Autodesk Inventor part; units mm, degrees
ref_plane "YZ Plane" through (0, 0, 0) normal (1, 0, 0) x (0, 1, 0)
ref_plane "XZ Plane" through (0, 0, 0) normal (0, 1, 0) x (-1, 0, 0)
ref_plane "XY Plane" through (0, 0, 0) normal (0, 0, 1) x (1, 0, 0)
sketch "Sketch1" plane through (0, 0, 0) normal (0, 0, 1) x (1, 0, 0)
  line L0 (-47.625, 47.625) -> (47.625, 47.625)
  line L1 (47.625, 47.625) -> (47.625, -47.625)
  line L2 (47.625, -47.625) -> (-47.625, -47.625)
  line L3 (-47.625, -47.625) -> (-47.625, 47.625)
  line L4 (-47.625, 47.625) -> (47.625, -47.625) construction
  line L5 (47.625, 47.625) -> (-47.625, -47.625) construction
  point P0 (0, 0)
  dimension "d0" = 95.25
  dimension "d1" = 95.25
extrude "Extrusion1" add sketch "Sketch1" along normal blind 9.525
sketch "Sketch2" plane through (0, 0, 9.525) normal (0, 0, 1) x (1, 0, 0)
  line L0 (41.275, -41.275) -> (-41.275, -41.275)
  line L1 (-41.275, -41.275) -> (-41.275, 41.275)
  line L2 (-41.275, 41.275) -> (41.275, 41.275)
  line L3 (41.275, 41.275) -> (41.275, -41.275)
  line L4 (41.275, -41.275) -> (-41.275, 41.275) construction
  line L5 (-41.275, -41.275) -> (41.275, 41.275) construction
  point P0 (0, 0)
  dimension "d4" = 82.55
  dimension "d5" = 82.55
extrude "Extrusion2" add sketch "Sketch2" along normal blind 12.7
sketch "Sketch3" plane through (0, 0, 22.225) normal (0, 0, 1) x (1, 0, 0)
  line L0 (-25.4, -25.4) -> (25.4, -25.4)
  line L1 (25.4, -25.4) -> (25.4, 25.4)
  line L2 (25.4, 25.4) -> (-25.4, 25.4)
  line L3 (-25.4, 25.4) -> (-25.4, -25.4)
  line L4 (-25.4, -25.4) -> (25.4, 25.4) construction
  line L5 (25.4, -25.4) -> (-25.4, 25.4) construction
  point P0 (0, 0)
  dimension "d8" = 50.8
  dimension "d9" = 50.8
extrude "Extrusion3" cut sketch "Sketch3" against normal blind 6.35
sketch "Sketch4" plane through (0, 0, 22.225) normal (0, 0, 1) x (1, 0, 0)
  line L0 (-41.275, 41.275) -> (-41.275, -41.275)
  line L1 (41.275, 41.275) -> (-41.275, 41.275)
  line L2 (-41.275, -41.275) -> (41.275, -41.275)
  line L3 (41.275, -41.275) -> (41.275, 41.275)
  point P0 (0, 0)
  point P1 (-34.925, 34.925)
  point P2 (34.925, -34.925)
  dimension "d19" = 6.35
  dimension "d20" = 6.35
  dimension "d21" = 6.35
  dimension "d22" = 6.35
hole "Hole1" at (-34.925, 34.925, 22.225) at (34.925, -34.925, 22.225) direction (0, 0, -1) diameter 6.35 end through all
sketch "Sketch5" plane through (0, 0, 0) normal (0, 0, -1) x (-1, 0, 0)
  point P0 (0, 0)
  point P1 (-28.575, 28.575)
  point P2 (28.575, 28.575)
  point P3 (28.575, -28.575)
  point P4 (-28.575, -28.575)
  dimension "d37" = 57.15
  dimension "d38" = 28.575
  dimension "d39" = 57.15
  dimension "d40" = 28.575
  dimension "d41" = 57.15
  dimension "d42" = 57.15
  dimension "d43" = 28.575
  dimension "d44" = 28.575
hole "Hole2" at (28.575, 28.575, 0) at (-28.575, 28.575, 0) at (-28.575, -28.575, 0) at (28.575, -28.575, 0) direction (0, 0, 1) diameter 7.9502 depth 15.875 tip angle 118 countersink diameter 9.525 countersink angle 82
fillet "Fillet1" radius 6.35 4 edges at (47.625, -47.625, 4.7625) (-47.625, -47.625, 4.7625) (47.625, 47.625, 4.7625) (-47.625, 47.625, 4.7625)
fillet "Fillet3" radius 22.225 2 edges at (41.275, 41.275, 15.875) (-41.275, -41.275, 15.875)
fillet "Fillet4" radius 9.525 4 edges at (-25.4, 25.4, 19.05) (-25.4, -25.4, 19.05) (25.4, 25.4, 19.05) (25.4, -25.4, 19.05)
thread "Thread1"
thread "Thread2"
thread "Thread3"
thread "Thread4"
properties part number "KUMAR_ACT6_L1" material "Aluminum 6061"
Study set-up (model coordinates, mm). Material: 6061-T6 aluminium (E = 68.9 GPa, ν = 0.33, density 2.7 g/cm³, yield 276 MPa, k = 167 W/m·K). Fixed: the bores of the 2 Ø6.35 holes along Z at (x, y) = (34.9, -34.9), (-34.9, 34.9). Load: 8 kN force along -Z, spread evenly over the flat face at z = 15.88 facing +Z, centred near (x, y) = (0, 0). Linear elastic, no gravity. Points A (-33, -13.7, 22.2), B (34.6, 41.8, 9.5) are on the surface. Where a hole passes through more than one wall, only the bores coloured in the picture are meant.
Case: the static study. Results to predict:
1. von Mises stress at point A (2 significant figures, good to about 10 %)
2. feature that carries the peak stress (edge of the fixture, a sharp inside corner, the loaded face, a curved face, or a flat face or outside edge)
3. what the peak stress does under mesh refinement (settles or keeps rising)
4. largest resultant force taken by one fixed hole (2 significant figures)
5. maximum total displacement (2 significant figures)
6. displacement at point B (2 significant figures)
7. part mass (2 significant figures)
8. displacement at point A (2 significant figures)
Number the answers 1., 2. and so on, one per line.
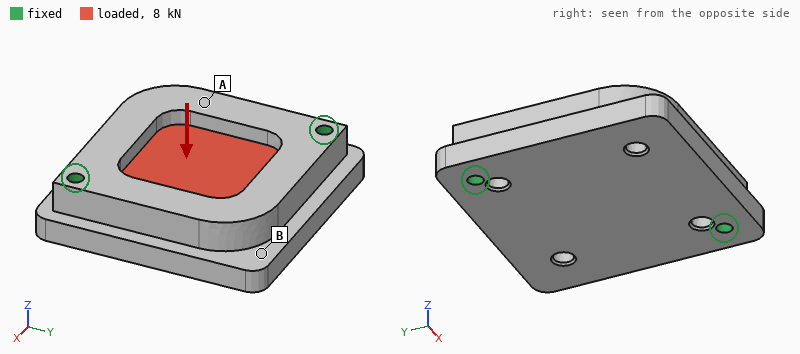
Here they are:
1. 14 MPa
2. edge of the fixture
3. keeps rising
4. 4.2 kN
5. 36 µm
6. 33 µm
7. 400 g
8. 27 µm
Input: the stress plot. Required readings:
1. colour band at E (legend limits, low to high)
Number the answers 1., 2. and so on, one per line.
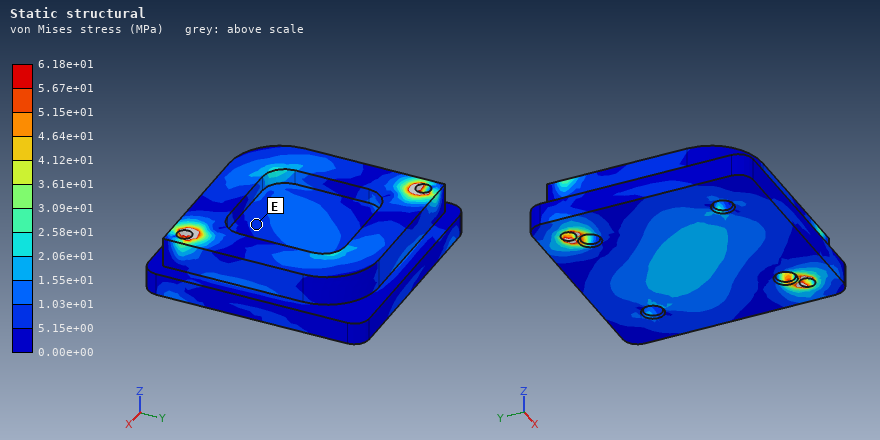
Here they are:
1. 5.15e+00 to 1.03e+01 MPa
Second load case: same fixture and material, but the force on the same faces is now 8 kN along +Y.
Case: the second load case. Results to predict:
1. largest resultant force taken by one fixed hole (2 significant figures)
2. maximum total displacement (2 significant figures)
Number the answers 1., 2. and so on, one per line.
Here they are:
1. 4.0 kN
2. 15 µm
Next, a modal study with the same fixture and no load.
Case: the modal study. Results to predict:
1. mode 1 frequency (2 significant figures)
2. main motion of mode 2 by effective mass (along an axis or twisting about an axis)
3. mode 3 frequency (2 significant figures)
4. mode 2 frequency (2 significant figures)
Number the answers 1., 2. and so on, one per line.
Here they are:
1. 3500 Hz
2. along Z
3. 9600 Hz
4. 4400 Hz
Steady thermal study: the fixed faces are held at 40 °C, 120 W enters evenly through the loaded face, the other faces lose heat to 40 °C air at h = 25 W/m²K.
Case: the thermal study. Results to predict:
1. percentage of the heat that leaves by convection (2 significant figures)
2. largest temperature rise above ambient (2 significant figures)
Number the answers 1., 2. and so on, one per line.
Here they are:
1. 5.9 %
2. 19 K
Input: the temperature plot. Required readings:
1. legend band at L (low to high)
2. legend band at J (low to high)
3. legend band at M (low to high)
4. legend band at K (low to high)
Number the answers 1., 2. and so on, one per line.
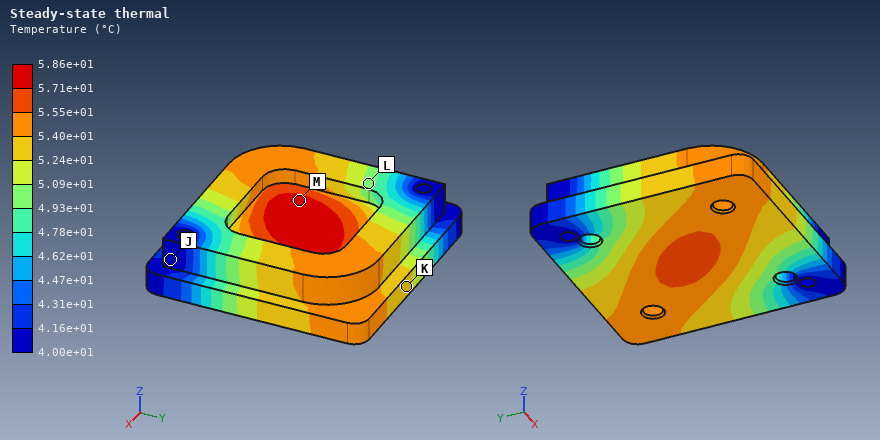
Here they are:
1. 4.93e+01 to 5.09e+01 °C
2. 4.00e+01 to 4.16e+01 °C
3. 5.71e+01 to 5.86e+01 °C
4. 5.24e+01 to 5.40e+01 °C
